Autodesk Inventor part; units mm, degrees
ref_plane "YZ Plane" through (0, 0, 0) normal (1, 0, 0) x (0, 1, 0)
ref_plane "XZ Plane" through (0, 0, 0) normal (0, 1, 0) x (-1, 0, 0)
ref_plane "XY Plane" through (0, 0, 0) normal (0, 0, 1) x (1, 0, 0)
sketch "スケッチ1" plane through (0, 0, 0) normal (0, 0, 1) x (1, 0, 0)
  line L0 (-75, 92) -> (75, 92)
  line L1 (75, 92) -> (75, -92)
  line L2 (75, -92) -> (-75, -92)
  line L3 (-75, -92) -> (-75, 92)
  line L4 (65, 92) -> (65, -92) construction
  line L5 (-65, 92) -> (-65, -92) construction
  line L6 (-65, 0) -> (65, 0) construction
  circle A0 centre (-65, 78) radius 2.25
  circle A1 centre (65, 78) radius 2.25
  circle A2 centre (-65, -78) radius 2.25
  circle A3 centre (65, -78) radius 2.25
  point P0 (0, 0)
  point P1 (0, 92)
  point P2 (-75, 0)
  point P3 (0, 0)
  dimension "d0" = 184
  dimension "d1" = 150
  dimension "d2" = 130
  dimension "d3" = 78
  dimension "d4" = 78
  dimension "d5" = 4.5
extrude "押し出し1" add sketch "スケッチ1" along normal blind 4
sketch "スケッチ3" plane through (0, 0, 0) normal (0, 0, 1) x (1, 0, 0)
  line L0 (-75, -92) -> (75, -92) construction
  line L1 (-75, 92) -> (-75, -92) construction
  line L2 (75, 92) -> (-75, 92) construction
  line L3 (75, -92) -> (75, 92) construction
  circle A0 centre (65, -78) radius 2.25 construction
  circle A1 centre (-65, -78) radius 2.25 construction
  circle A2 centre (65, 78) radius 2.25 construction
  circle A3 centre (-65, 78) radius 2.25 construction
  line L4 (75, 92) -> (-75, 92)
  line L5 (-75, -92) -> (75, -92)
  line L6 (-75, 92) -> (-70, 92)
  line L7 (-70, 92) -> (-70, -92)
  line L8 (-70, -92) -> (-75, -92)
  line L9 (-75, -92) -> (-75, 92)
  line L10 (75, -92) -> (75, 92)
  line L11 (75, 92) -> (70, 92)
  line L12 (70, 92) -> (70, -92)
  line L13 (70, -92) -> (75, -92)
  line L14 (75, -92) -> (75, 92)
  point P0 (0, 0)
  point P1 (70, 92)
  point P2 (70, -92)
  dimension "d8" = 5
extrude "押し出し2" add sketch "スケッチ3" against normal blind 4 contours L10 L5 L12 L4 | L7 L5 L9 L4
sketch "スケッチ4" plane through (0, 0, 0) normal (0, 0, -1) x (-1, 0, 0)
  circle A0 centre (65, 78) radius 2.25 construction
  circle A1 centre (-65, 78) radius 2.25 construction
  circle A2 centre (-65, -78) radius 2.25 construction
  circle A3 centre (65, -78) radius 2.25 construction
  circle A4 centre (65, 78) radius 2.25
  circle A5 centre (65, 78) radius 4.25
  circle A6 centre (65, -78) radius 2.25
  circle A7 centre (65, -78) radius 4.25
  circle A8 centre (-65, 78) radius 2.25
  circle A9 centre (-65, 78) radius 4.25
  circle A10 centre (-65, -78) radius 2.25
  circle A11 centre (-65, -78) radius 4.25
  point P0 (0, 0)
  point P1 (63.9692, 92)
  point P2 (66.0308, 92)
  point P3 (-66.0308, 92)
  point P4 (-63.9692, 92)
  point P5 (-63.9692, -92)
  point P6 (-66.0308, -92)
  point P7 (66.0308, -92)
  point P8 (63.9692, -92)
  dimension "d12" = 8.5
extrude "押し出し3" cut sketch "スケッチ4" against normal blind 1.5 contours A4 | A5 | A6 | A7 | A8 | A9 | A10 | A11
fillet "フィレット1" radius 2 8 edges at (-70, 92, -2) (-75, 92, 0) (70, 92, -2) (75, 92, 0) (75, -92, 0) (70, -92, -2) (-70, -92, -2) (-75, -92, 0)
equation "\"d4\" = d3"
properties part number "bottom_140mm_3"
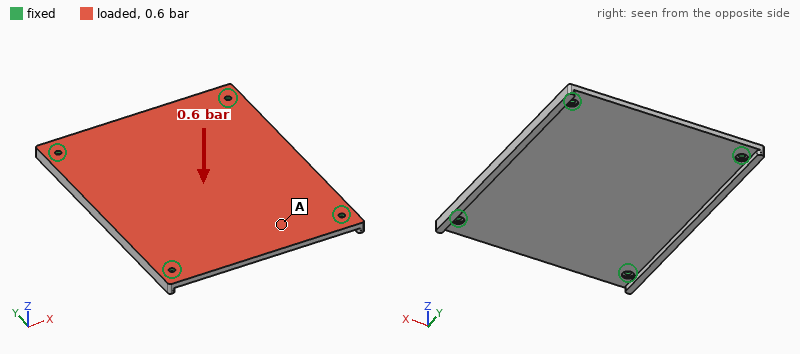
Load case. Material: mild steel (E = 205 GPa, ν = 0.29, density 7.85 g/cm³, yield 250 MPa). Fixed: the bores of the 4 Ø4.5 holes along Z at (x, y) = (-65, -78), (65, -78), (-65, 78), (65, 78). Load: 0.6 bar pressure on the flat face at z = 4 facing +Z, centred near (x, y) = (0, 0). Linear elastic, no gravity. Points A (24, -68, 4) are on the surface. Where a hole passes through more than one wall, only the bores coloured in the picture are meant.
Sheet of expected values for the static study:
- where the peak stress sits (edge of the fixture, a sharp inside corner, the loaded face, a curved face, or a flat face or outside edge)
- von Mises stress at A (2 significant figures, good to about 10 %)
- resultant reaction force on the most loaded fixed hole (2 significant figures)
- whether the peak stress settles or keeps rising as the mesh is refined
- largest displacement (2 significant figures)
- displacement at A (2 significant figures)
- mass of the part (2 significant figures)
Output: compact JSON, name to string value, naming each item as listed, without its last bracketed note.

{"where the peak stress sits": "edge of the fixture", "von Mises stress at A": "17 MPa", "resultant reaction force on the most loaded fixed hole": "780 N", "whether the peak stress settles or keeps rising as the mesh is refined": "keeps rising", "largest displacement": "0.18 mm", "displacement at A": "0.085 mm", "mass of the part": "920 g"}
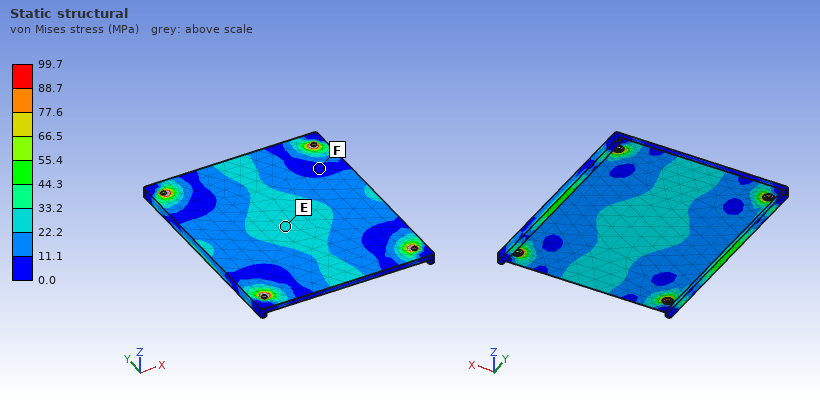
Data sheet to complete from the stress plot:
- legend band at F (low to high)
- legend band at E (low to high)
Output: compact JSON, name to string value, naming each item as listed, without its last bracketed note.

{"legend band at F": "0.0 to 11.1 MPa", "legend band at E": "22.2 to 33.2 MPa"}
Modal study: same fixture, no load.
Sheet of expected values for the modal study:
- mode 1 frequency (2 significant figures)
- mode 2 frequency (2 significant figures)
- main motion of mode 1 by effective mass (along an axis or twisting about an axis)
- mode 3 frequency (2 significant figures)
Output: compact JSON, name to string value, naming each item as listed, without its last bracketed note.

{"mode 1 frequency": "630 Hz", "mode 2 frequency": "1100 Hz", "main motion of mode 1 by effective mass": "along Z", "mode 3 frequency": "1100 Hz"}
